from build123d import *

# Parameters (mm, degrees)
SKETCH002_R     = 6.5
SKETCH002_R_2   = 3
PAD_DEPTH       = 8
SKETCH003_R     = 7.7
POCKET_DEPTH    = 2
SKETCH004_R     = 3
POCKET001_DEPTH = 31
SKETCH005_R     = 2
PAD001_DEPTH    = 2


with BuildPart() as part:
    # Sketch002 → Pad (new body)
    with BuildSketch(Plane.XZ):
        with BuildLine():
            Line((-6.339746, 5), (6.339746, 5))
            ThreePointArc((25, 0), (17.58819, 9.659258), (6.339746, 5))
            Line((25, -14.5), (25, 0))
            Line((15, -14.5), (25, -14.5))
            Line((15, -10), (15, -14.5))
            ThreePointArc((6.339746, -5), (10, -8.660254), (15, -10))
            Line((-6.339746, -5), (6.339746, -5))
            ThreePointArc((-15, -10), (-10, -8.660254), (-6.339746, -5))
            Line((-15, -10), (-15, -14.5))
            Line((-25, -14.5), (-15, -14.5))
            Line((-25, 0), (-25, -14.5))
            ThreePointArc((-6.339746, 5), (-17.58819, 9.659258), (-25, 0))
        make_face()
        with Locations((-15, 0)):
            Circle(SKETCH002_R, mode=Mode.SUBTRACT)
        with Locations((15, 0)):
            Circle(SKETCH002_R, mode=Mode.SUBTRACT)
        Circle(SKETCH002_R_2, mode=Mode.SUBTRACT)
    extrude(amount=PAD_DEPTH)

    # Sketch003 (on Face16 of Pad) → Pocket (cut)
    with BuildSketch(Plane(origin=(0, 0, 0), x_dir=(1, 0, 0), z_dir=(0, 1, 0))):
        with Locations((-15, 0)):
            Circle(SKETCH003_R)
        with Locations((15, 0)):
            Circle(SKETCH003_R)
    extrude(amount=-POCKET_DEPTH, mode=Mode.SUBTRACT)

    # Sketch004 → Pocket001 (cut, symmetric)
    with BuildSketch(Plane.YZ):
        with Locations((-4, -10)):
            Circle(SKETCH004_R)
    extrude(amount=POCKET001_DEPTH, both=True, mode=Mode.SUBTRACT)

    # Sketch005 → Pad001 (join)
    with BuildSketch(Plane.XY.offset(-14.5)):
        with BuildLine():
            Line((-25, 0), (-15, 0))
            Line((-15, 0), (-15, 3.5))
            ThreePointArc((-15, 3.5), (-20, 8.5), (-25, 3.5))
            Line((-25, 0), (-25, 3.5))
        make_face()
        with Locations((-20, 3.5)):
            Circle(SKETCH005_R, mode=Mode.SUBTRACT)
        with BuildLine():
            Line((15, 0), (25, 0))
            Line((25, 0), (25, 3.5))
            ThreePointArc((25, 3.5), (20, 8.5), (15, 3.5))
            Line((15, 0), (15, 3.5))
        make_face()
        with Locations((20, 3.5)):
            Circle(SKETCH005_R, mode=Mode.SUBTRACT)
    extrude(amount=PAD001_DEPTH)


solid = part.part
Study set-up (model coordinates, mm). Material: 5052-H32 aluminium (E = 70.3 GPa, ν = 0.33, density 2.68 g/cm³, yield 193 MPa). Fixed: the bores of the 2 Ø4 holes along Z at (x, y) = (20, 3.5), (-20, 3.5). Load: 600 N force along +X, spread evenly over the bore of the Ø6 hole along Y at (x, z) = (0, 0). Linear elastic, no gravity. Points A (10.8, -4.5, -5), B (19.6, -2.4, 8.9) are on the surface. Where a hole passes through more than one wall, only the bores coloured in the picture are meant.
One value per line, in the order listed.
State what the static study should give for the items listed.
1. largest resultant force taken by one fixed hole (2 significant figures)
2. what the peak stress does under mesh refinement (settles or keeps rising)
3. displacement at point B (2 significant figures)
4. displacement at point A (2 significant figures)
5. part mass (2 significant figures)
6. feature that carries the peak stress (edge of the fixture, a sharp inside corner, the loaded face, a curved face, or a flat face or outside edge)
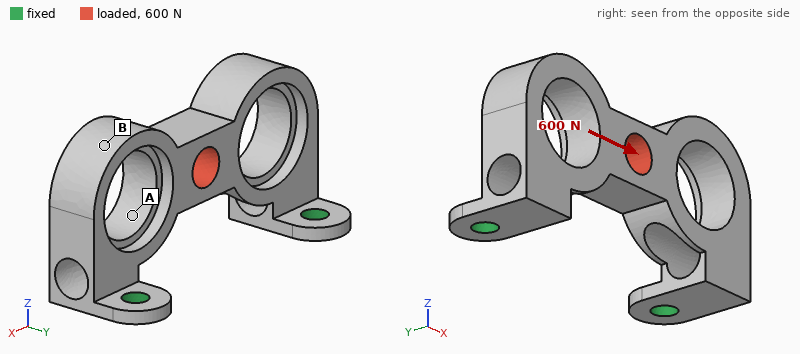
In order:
350 N
keeps rising
35 µm
20 µm
11 g
a sharp inside corner
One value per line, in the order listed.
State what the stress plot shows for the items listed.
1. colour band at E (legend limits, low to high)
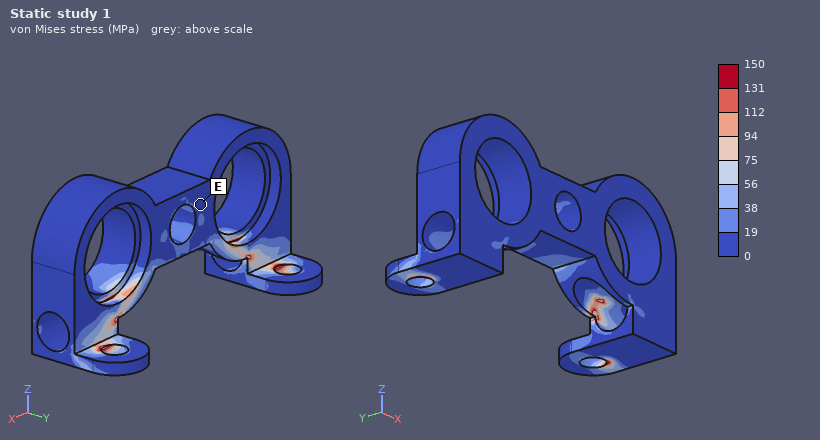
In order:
0 to 19 MPa
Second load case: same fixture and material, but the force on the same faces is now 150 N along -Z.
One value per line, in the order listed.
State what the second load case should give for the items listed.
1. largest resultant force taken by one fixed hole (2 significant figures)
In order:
97 N
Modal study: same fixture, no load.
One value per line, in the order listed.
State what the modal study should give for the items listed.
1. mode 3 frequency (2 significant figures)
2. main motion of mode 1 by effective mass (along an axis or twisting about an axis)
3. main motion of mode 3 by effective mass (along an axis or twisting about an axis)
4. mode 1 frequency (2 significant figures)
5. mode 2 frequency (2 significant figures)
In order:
8600 Hz
along Y
along X
1600 Hz
5300 Hz
